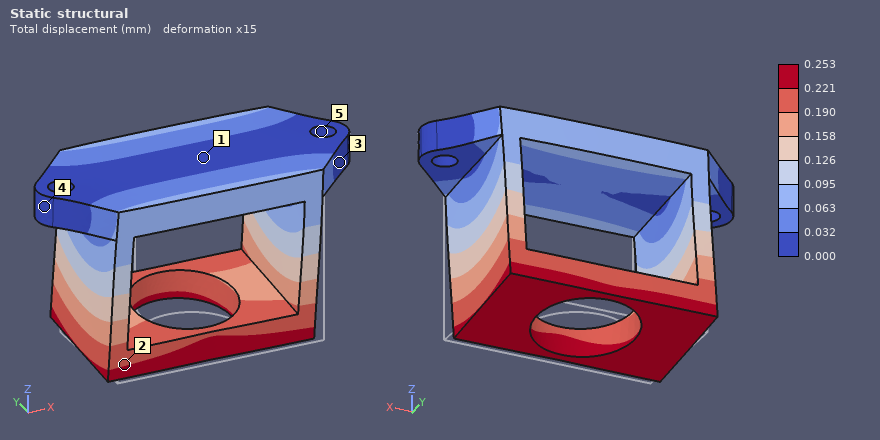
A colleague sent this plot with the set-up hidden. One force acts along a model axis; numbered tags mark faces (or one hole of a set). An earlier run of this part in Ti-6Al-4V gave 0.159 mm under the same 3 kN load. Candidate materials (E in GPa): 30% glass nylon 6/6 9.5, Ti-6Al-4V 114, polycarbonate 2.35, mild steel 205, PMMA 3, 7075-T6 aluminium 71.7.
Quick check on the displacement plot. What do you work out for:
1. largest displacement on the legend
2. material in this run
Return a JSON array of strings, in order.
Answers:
["0.253 mm", "7075-T6 aluminium"]
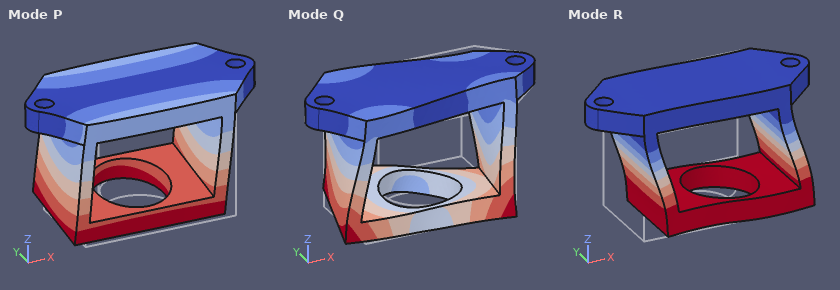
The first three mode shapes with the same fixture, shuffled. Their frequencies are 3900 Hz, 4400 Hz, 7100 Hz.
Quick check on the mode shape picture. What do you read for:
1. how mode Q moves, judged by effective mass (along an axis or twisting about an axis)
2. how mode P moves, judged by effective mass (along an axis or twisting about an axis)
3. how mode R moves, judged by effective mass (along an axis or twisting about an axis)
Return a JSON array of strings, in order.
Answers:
["twisting about Z", "along Y", "along X"]
